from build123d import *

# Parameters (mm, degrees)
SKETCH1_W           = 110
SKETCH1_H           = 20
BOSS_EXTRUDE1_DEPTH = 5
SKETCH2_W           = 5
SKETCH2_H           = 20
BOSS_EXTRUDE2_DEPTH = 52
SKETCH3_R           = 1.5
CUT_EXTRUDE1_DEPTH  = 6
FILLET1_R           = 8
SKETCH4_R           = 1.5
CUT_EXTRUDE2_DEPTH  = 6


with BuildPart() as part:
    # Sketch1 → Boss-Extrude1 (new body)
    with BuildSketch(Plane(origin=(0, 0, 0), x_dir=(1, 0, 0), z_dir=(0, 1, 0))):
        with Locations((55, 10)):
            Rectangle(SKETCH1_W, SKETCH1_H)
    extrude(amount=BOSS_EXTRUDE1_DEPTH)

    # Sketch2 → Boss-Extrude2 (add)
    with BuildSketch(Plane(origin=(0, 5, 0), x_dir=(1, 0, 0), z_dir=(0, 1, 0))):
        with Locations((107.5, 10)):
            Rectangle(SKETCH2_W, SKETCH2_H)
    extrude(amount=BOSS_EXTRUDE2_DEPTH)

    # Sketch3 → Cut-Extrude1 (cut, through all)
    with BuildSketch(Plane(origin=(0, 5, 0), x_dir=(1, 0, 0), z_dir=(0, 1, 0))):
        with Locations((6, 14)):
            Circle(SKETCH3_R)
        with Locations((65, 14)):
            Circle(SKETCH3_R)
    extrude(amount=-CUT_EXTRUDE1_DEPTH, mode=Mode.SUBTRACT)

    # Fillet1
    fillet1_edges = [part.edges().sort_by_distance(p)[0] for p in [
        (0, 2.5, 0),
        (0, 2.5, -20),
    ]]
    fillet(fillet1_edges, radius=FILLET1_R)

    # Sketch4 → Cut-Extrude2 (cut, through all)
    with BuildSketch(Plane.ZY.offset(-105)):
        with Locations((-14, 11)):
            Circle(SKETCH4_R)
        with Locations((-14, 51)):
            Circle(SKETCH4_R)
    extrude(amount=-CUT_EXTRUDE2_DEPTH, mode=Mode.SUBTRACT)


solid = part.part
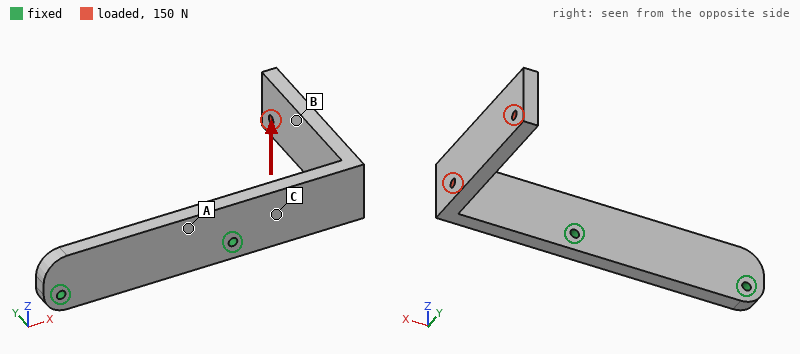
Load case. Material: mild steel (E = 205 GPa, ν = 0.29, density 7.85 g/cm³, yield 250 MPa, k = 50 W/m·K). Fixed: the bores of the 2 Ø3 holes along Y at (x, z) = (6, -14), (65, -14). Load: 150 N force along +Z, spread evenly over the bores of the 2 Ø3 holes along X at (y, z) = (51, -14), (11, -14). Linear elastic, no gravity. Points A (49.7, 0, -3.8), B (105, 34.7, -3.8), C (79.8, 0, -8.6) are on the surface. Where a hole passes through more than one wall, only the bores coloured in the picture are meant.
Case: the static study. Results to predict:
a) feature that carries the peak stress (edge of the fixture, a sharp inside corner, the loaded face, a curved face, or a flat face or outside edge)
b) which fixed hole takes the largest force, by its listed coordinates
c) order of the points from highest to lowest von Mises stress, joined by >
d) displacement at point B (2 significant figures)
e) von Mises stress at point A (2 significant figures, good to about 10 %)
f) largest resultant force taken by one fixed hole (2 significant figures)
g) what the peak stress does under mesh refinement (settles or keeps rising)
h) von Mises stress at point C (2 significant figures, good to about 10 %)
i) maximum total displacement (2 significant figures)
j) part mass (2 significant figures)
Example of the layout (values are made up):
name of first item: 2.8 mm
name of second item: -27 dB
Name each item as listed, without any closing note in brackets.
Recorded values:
feature that carries the peak stress: edge of the fixture
which fixed hole takes the largest force, by its listed coordinates: (65, -14)
order of the points from highest to lowest von Mises stress, joined by >: C > A > B
displacement at point B: 0.12 mm
von Mises stress at point A: 13 MPa
largest resultant force taken by one fixed hole: 300 N
what the peak stress does under mesh refinement: keeps rising
von Mises stress at point C: 45 MPa
maximum total displacement: 0.19 mm
part mass: 120 g
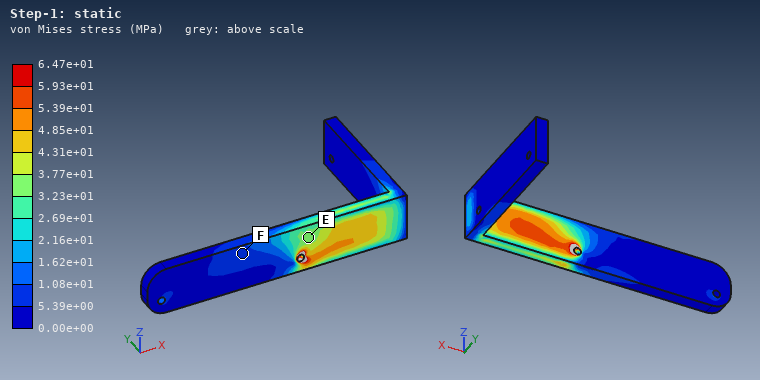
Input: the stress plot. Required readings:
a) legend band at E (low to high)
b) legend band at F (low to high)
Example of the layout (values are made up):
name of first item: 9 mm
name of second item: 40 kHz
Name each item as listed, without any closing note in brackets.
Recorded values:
legend band at E: 3.23e+01 to 3.77e+01 MPa
legend band at F: 5.39e+00 to 1.08e+01 MPa
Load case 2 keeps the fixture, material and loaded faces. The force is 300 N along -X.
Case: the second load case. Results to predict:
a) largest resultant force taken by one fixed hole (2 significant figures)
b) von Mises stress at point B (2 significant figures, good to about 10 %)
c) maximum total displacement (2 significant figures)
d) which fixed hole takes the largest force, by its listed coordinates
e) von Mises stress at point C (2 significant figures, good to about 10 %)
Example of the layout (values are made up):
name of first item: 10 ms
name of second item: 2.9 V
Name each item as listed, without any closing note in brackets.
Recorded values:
largest resultant force taken by one fixed hole: 290 N
von Mises stress at point B: 30 MPa
maximum total displacement: 0.67 mm
which fixed hole takes the largest force, by its listed coordinates: (65, -14)
von Mises stress at point C: 97 MPa
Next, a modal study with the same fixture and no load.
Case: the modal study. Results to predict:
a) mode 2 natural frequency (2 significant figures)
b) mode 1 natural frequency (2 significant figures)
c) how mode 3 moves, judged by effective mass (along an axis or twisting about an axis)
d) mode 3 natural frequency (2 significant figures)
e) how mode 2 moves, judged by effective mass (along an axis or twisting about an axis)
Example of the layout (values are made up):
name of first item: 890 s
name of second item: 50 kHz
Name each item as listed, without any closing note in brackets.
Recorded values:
mode 2 natural frequency: 840 Hz
mode 1 natural frequency: 570 Hz
how mode 3 moves, judged by effective mass: along Y
mode 3 natural frequency: 1600 Hz
how mode 2 moves, judged by effective mass: along Z
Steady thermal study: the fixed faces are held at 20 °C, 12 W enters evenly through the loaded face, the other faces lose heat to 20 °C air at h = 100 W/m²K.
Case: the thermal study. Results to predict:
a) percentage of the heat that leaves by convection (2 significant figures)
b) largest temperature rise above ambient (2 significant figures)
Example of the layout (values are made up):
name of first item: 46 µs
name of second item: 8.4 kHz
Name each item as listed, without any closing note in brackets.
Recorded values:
percentage of the heat that leaves by convection: 87 %
largest temperature rise above ambient: 45 K
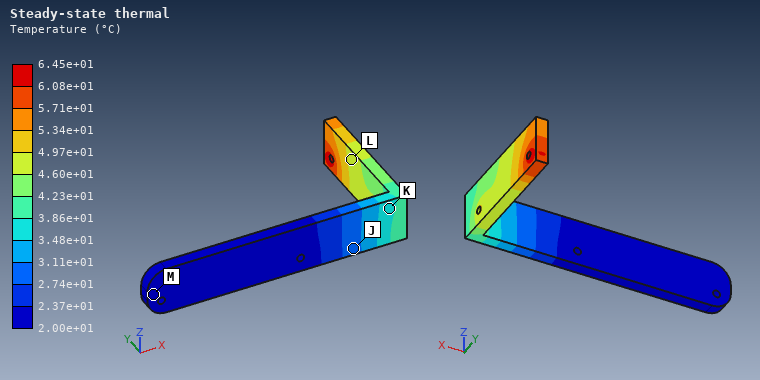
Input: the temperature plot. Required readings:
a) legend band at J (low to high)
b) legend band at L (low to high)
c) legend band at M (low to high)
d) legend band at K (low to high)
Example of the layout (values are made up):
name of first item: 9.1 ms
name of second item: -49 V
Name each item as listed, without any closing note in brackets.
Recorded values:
legend band at J: 2.74e+01 to 3.11e+01 °C
legend band at L: 4.60e+01 to 4.97e+01 °C
legend band at M: 2.00e+01 to 2.37e+01 °C
legend band at K: 3.48e+01 to 3.86e+01 °C
